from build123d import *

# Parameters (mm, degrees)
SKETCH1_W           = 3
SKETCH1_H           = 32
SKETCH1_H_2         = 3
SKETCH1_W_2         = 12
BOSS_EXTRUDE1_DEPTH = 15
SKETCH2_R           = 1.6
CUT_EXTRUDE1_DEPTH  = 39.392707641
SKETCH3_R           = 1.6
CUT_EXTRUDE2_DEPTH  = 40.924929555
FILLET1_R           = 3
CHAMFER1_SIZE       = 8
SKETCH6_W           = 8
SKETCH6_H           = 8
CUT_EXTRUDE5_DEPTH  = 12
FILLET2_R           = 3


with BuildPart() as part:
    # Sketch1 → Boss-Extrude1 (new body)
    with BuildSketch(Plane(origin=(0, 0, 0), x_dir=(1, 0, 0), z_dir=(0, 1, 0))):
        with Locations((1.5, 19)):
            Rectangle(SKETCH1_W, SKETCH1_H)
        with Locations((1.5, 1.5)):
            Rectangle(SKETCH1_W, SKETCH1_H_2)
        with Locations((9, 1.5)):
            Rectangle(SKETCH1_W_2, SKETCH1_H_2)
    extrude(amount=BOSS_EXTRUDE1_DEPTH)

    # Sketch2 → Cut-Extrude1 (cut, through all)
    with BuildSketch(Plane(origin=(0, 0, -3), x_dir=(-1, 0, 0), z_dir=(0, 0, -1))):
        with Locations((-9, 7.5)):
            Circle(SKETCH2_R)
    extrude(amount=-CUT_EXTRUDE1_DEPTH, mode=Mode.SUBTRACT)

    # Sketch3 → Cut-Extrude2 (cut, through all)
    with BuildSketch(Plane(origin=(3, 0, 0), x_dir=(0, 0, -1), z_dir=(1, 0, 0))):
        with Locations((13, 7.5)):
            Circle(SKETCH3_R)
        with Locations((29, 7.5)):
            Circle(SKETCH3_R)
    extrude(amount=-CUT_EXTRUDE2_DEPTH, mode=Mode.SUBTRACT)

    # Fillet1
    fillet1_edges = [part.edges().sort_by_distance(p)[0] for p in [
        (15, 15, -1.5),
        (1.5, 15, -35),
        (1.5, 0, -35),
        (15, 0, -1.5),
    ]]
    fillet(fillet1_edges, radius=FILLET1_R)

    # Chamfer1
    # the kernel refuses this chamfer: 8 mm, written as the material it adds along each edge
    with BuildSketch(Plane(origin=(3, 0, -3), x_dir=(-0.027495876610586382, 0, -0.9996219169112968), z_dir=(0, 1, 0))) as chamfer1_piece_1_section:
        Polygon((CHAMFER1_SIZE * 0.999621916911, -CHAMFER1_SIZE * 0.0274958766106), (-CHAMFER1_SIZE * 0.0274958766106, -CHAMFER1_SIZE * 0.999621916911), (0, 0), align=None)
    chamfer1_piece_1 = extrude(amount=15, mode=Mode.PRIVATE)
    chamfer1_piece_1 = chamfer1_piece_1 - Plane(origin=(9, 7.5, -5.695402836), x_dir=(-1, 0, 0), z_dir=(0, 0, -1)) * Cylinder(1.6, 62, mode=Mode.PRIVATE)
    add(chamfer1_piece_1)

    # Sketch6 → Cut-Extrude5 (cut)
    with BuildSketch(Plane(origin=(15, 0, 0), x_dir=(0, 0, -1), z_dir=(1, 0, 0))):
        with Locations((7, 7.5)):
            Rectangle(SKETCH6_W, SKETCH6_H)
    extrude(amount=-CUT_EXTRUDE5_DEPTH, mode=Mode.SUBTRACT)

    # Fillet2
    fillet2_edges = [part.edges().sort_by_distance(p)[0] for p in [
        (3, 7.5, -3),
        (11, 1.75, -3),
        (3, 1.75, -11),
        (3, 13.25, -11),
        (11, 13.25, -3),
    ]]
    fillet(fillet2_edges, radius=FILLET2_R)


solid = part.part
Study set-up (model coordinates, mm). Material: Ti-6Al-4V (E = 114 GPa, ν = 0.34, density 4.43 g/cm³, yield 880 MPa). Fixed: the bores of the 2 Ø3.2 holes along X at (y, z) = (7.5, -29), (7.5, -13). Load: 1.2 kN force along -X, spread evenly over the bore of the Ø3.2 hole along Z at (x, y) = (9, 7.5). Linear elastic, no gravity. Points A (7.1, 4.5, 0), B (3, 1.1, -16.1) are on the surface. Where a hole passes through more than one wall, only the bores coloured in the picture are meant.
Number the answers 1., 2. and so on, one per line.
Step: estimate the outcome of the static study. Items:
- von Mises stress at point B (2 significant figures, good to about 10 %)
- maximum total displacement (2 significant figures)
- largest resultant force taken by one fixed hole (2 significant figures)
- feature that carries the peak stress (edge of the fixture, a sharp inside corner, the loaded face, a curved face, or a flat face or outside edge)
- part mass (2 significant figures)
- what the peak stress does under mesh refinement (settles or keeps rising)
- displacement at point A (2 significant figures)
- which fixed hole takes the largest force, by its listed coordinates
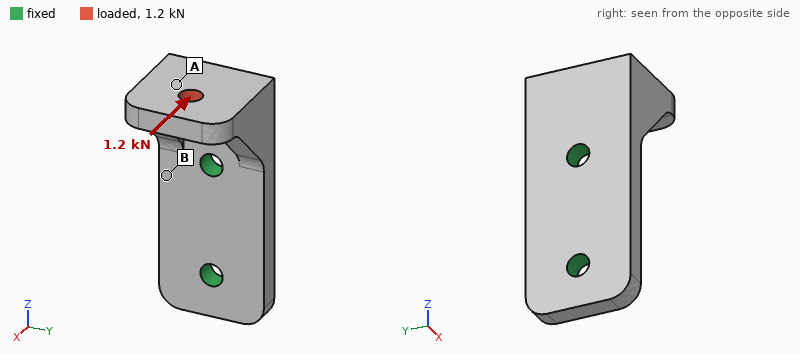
1. 120 MPa
2. 0.22 mm
3. 1.4 kN
4. edge of the fixture
5. 10 g
6. keeps rising
7. 0.16 mm
8. (7.5, -13)
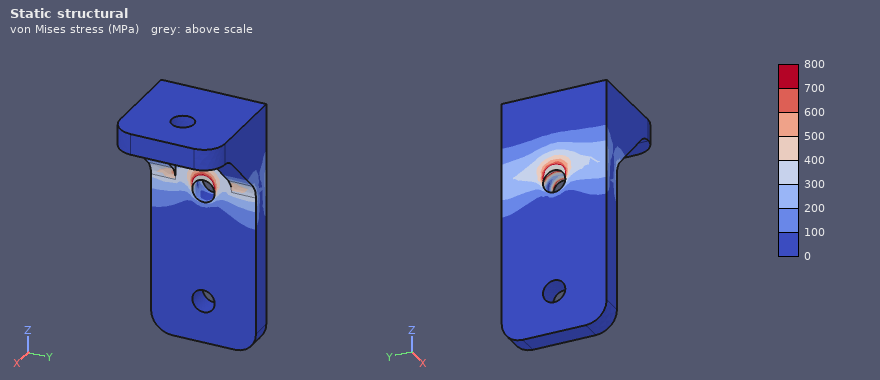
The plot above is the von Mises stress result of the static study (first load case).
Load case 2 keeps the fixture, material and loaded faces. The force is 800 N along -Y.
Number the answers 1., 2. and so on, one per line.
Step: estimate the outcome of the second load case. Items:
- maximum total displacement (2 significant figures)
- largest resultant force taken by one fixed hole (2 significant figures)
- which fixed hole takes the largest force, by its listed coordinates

1. 93 µm
2. 1.2 kN
3. (7.5, -13)
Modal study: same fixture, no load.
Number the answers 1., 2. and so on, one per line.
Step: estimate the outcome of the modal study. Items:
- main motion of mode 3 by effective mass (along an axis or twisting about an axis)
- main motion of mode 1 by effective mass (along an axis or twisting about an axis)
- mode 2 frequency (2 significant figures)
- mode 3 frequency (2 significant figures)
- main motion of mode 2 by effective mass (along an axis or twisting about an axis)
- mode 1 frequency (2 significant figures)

1. along Y
2. along X
3. 9500 Hz
4. 20 kHz
5. along Y
6. 6700 Hz
